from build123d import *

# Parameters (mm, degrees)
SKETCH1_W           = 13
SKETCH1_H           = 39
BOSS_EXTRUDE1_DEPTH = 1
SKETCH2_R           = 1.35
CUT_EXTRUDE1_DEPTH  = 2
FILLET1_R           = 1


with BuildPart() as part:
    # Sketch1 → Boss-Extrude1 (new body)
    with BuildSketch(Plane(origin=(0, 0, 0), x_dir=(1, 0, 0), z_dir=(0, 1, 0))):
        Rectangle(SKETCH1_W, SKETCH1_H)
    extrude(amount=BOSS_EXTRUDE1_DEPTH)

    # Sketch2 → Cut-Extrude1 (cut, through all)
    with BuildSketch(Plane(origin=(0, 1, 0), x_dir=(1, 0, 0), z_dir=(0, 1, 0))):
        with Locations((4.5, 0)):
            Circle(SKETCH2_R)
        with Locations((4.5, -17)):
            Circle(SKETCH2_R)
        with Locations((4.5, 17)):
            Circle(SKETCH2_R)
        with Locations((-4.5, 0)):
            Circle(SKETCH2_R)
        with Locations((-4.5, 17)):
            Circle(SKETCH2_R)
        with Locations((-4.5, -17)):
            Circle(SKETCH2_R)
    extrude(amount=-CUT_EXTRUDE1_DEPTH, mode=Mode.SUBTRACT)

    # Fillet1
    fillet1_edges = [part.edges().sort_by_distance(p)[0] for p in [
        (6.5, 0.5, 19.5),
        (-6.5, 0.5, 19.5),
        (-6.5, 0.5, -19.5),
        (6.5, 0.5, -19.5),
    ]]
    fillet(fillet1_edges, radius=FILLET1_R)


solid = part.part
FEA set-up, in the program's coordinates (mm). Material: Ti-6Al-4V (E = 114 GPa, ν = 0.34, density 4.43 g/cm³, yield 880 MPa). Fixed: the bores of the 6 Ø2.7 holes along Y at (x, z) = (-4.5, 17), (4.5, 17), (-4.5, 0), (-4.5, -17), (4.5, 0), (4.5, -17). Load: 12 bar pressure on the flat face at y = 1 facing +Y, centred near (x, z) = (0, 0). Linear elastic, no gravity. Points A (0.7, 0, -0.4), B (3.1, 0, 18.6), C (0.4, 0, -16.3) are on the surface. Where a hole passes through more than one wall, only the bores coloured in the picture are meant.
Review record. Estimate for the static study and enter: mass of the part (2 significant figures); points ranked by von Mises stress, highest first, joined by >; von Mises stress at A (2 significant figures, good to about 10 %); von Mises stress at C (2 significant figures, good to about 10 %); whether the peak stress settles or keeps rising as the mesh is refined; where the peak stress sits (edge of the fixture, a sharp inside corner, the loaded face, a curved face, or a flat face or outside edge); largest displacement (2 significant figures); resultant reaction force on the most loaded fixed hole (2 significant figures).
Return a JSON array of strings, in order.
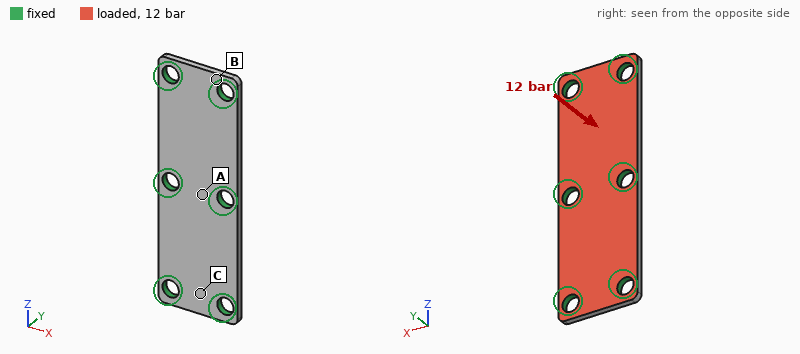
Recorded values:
["2.1 g", "A > C > B", "65 MPa", "43 MPa", "keeps rising", "edge of the fixture", "19 µm", "130 N"]
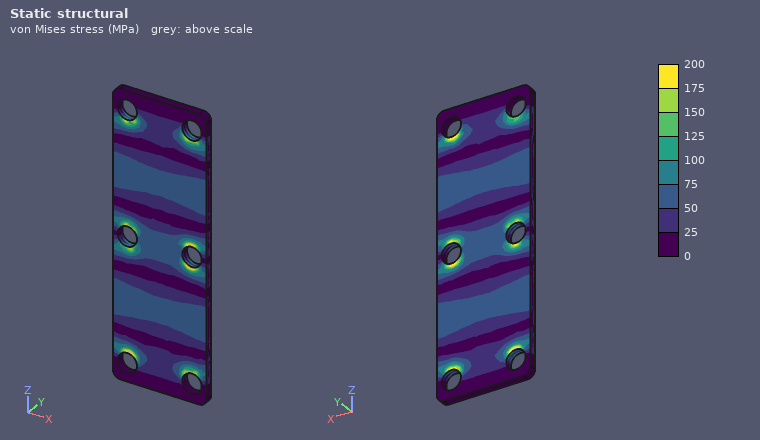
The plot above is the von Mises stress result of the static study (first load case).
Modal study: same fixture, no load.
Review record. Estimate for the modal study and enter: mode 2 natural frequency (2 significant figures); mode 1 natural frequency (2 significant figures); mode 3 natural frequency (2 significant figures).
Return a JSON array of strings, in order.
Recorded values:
["22 kHz", "22 kHz", "29 kHz"]
